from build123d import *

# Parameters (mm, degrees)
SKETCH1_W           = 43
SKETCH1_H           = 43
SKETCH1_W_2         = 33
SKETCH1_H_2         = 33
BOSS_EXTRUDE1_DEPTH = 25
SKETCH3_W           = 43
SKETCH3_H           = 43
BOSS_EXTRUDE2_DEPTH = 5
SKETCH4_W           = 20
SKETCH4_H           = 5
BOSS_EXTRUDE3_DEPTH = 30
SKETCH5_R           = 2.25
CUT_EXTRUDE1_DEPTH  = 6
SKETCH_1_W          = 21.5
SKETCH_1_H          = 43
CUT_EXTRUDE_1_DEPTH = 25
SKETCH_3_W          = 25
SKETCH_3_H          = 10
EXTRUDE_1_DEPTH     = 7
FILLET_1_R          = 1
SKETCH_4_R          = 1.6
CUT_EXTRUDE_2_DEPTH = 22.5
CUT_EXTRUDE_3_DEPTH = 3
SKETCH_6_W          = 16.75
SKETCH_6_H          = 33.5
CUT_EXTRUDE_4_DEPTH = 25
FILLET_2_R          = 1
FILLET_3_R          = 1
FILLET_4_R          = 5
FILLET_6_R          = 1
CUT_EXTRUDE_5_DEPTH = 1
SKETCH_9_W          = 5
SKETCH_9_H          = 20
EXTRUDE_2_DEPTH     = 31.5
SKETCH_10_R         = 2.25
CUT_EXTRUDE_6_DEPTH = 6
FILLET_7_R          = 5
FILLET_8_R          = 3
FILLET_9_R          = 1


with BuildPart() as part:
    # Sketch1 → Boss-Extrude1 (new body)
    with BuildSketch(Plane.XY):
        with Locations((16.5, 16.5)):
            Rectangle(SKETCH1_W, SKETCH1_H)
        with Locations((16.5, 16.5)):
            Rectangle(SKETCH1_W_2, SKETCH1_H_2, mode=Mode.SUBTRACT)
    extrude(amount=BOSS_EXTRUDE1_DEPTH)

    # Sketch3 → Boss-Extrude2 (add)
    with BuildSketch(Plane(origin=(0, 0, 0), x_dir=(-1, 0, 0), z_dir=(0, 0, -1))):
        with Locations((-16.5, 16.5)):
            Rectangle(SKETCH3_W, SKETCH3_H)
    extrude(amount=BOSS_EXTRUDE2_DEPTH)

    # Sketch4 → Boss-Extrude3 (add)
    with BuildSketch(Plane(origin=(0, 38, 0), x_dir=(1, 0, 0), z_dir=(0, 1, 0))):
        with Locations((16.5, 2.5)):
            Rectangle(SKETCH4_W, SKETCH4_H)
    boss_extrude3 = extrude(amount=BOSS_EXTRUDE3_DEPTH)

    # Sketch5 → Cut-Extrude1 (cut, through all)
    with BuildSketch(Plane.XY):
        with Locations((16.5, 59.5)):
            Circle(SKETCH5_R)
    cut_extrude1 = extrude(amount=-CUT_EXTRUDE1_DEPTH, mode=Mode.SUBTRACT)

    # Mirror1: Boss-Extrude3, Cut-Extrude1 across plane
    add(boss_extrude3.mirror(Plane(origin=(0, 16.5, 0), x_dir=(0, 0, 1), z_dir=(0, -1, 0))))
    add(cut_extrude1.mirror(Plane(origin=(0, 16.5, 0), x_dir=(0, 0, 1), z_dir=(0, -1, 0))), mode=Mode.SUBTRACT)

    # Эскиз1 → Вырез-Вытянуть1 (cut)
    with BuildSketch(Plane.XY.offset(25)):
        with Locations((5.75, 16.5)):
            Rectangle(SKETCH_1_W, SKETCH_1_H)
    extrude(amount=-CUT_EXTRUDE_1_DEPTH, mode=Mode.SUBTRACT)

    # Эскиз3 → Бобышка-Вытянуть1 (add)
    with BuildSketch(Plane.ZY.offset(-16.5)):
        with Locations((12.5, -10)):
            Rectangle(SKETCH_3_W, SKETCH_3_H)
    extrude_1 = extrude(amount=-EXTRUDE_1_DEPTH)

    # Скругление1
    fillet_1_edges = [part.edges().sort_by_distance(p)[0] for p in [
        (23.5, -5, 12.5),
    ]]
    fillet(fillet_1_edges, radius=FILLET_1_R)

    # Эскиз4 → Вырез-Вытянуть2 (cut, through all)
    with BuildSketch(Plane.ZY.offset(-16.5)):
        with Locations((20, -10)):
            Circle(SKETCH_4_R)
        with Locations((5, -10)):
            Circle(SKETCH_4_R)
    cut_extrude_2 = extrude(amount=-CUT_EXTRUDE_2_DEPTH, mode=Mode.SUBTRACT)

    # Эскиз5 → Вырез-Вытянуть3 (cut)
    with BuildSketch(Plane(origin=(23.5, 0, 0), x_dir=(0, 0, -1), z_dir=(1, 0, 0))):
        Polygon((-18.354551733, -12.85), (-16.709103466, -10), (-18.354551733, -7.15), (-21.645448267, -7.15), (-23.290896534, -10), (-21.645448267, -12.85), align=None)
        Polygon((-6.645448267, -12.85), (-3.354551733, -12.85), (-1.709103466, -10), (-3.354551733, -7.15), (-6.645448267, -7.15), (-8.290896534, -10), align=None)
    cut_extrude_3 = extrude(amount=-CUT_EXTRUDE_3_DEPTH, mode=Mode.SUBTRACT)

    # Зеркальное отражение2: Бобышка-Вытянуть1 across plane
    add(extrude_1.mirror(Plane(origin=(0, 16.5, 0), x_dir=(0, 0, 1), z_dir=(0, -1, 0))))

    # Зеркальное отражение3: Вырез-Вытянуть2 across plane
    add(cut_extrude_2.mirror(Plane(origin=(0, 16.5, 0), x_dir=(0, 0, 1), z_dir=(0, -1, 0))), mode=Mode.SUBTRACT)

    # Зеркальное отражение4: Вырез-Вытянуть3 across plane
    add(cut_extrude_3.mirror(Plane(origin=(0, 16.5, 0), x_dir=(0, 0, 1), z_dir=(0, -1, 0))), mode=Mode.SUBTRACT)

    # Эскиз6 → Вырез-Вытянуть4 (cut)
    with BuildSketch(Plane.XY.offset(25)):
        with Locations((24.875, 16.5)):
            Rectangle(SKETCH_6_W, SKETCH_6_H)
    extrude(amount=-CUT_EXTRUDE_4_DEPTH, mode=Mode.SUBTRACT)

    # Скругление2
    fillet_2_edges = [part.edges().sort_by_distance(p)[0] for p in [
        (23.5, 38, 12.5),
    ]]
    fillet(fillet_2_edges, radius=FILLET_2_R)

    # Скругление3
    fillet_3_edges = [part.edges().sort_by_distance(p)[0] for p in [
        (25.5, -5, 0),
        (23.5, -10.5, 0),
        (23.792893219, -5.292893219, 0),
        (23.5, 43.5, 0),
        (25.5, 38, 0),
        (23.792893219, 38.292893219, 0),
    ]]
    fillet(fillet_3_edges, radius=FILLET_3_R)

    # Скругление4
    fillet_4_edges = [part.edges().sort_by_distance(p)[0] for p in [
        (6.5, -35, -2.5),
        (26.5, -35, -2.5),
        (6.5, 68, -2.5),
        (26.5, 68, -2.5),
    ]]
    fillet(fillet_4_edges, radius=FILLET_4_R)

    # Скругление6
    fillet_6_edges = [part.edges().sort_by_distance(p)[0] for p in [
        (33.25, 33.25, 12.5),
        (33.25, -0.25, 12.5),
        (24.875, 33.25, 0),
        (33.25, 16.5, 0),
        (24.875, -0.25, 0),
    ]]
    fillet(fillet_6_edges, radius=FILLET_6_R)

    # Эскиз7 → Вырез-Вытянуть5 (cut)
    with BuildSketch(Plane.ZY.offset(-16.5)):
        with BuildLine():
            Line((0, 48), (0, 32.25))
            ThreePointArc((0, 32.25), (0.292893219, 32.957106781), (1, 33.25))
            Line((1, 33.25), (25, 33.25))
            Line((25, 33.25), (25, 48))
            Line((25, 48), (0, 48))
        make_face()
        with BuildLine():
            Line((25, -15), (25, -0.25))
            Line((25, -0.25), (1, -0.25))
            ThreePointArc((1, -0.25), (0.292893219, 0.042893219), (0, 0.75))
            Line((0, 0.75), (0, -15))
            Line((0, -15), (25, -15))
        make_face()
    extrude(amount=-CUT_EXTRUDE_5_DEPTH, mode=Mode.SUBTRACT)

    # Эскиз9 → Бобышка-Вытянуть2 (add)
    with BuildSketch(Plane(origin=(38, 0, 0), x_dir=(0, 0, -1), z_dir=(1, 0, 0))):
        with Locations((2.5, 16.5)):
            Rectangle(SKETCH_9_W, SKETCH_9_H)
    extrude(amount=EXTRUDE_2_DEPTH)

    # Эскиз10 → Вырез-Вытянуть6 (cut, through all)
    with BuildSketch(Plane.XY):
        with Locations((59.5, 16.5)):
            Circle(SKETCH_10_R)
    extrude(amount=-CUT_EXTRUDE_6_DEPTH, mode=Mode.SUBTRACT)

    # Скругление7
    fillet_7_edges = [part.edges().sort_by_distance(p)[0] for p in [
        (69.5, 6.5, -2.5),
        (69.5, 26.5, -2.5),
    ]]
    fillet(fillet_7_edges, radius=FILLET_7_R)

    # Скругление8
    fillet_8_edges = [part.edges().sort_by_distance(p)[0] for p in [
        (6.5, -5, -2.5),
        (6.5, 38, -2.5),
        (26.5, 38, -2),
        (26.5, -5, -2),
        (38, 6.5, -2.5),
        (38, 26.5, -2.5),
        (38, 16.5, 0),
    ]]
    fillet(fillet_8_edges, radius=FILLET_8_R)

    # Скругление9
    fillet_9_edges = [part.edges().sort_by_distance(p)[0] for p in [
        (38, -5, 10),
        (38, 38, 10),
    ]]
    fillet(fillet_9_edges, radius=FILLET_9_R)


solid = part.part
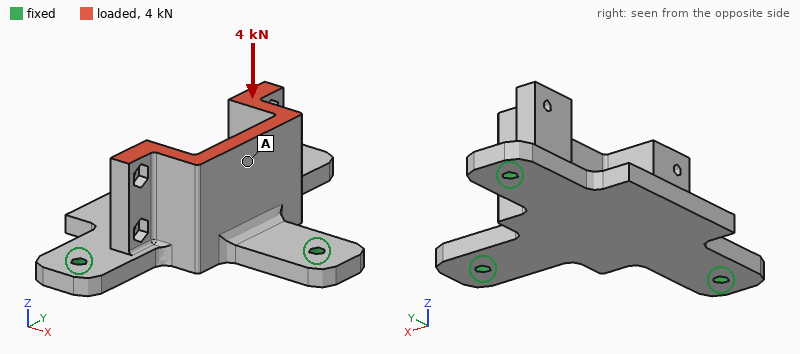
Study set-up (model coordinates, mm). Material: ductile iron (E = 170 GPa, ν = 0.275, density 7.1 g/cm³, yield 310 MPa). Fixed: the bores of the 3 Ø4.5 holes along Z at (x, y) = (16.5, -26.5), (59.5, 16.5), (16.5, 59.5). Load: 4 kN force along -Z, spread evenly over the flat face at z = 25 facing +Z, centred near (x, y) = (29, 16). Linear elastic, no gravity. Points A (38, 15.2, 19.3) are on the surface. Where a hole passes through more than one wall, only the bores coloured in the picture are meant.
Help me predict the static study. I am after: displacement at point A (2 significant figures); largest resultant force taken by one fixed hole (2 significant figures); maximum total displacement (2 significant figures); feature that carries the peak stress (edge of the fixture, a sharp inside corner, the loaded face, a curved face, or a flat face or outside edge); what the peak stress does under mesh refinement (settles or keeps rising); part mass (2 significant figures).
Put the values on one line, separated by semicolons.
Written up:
45 µm; 1.4 kN; 47 µm; edge of the fixture; keeps rising; 210 g
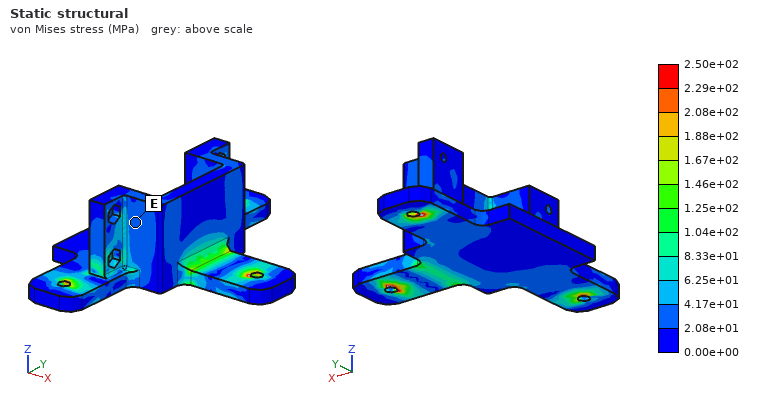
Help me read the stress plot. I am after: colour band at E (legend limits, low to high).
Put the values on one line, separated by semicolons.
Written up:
2.08e+01 to 4.17e+01 MPa
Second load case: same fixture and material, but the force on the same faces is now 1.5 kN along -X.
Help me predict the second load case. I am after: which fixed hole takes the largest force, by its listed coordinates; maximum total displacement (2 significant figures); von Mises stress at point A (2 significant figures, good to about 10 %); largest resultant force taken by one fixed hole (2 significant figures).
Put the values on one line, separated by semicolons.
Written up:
(59.5, 16.5); 58 µm; 18 MPa; 1.4 kN
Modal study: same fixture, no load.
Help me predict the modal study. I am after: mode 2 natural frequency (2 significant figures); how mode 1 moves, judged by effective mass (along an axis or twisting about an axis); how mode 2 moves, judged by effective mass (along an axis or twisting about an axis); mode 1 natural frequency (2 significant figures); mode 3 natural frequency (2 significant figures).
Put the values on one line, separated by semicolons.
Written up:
4300 Hz; along Z; along Z; 3200 Hz; 5600 Hz
